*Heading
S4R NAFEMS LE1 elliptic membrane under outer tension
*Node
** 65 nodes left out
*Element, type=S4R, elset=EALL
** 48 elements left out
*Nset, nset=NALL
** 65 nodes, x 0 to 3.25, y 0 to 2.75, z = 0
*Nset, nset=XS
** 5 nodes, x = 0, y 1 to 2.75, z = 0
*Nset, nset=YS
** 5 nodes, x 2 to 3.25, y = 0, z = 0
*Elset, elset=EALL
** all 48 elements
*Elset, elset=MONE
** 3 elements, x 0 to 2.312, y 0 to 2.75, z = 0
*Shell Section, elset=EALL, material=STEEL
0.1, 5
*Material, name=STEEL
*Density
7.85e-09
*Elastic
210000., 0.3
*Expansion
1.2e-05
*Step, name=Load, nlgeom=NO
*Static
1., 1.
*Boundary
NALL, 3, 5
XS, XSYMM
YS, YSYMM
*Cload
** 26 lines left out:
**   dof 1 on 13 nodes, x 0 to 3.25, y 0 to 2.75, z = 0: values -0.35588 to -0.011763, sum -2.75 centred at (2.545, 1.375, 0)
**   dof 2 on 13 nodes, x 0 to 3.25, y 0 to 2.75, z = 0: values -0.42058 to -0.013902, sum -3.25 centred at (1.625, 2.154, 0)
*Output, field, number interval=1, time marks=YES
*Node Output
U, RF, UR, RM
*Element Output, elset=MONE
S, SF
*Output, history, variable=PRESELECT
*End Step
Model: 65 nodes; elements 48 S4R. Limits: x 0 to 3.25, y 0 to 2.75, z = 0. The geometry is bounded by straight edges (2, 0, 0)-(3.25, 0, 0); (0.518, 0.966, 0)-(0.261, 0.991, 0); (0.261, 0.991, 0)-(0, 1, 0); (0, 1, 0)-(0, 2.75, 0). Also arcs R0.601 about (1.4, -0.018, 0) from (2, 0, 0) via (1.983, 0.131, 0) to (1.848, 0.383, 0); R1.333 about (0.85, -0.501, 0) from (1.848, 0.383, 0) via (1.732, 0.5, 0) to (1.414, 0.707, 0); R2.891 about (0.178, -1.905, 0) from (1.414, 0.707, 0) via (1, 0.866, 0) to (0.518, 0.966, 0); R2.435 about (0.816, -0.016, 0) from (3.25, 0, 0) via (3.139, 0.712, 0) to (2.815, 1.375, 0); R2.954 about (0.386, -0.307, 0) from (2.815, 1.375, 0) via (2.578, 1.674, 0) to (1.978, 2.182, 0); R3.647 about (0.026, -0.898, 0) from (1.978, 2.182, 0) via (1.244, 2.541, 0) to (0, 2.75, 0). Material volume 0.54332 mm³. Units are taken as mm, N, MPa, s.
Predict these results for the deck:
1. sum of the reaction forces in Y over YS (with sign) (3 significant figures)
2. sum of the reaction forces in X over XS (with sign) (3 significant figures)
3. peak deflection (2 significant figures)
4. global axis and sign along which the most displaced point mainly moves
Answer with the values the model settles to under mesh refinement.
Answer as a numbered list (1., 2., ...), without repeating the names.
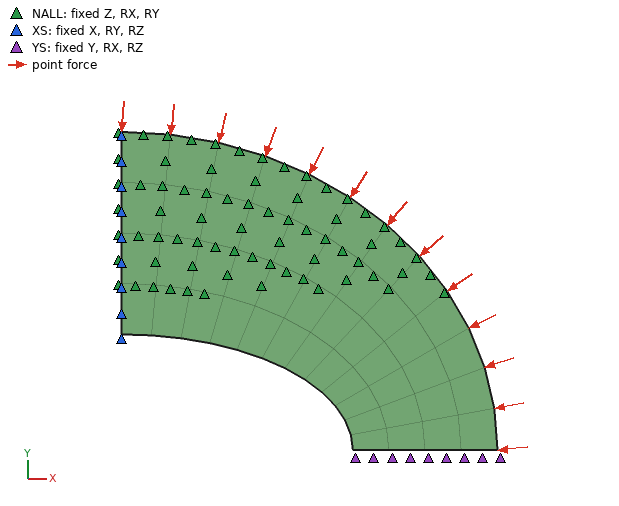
1. 3.25 N
2. 2.75 N
3. 5.6e-04 mm
4. -Y
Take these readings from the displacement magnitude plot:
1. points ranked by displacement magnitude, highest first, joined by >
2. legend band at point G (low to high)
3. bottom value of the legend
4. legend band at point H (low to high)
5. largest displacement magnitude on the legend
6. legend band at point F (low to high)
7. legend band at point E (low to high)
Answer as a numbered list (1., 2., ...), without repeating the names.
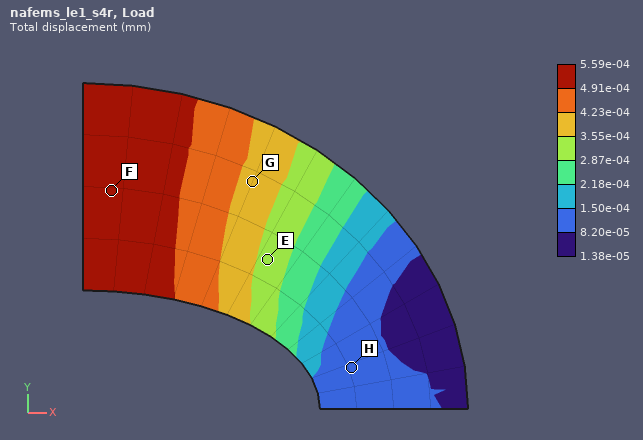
1. F > G > E > H
2. 3.55e-04 to 4.23e-04 mm
3. 1.38e-05 mm
4. 8.20e-05 to 1.50e-04 mm
5. 5.59e-04 mm
6. 4.91e-04 to 5.59e-04 mm
7. 2.87e-04 to 3.55e-04 mm
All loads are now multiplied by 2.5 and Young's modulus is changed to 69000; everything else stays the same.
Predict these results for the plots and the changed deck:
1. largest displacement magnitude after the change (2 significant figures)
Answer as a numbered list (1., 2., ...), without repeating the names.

1. 0.0043 mm
